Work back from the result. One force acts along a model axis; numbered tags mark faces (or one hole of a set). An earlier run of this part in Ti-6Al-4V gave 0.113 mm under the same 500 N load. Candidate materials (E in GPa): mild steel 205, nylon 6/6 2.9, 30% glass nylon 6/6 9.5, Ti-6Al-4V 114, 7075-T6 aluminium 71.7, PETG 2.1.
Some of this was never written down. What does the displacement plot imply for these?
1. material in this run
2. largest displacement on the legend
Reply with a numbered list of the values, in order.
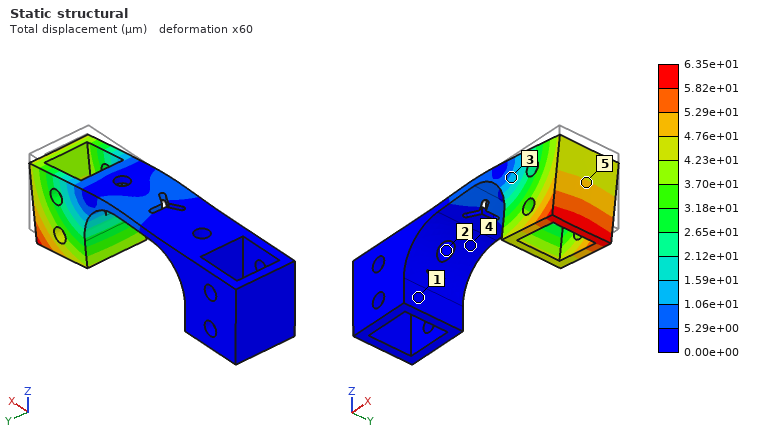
1. mild steel
2. 6.35e+01 µm
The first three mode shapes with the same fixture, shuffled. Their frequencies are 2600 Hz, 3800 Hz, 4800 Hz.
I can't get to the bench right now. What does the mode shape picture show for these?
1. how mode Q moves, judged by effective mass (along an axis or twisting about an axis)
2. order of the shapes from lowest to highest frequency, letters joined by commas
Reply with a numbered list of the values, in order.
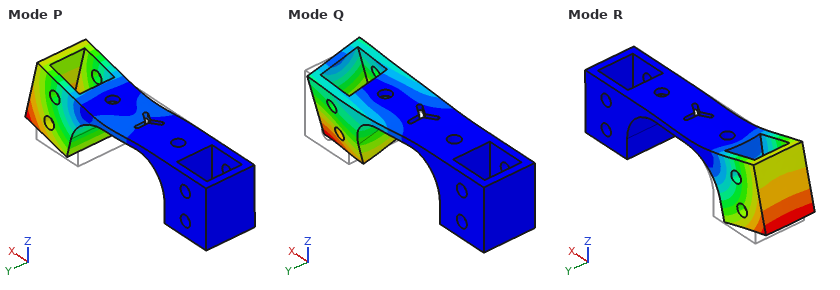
1. along Y
2. P, Q, R
